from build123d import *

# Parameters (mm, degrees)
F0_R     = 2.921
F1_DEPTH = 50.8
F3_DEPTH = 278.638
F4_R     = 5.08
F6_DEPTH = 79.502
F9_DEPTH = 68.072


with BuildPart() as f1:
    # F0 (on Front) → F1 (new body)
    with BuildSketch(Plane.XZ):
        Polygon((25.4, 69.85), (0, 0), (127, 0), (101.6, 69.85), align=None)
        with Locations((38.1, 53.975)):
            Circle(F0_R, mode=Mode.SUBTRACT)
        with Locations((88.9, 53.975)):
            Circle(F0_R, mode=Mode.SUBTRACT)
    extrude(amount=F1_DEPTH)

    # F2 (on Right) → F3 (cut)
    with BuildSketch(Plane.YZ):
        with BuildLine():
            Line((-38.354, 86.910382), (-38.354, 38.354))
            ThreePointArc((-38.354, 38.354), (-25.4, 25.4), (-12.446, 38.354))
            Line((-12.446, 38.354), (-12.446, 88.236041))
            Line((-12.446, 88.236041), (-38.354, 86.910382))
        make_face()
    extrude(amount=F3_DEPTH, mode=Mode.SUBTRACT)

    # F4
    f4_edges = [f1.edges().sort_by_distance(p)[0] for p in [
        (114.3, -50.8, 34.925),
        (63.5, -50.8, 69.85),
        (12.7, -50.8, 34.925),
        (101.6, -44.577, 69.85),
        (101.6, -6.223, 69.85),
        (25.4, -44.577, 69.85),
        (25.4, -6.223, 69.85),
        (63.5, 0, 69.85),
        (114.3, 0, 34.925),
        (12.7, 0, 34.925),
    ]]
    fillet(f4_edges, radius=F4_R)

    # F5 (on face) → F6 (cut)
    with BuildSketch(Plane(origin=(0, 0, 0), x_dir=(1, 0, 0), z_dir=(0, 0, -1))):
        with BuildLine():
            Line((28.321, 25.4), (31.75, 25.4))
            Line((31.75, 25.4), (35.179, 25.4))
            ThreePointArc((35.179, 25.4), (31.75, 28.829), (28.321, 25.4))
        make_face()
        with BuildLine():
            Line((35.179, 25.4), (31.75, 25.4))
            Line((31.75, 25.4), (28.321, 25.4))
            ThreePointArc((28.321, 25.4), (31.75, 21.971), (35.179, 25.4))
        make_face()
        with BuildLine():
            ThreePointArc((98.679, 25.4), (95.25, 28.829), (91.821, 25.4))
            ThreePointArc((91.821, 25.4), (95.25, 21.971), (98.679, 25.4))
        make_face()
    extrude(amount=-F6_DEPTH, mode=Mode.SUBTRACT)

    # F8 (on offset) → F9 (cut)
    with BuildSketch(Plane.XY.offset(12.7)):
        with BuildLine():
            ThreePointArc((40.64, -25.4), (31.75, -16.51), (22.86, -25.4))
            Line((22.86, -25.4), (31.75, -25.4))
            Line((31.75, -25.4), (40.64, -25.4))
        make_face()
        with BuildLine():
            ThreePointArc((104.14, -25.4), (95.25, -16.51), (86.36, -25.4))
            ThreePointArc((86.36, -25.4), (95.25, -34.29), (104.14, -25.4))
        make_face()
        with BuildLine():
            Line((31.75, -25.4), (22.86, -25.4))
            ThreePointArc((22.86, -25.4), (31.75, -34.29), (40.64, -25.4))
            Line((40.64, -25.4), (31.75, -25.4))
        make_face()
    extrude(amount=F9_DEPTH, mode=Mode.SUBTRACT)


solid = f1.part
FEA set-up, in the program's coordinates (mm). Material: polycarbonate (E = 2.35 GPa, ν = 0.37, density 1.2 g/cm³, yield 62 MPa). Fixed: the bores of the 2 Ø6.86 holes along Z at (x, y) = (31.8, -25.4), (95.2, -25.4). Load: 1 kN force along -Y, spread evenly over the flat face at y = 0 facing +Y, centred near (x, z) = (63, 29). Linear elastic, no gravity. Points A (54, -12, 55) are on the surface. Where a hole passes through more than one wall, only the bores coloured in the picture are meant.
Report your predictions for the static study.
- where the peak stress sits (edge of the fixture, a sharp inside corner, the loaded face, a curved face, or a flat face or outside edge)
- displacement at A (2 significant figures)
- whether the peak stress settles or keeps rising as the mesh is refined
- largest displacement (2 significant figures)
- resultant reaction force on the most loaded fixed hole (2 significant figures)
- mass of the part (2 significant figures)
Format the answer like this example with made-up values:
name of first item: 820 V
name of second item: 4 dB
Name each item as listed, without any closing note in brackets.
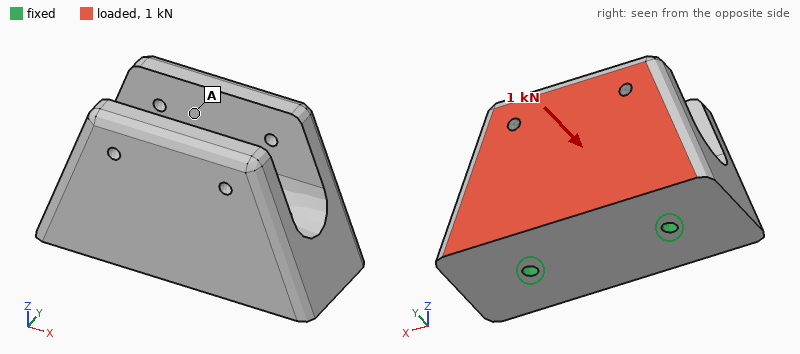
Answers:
where the peak stress sits: edge of the fixture
displacement at A: 0.37 mm
whether the peak stress settles or keeps rising as the mesh is refined: keeps rising
largest displacement: 0.51 mm
resultant reaction force on the most loaded fixed hole: 500 N
mass of the part: 300 g
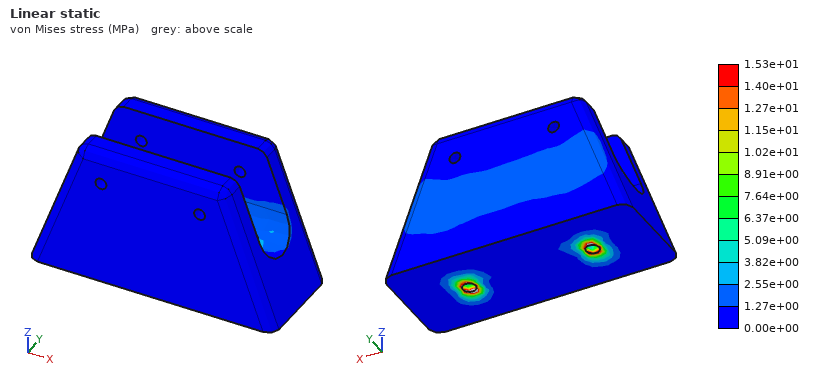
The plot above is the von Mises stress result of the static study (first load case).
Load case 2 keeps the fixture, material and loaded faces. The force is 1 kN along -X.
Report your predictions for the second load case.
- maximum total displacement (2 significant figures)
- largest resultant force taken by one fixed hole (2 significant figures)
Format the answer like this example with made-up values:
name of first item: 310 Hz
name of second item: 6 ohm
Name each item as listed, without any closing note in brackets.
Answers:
maximum total displacement: 64 µm
largest resultant force taken by one fixed hole: 710 N
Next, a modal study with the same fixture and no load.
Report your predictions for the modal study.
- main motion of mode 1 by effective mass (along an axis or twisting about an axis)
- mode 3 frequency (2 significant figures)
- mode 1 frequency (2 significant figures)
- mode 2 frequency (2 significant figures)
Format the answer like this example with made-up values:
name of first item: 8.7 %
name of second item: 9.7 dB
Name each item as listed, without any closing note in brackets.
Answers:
main motion of mode 1 by effective mass: along Y
mode 3 frequency: 1500 Hz
mode 1 frequency: 570 Hz
mode 2 frequency: 1400 Hz
